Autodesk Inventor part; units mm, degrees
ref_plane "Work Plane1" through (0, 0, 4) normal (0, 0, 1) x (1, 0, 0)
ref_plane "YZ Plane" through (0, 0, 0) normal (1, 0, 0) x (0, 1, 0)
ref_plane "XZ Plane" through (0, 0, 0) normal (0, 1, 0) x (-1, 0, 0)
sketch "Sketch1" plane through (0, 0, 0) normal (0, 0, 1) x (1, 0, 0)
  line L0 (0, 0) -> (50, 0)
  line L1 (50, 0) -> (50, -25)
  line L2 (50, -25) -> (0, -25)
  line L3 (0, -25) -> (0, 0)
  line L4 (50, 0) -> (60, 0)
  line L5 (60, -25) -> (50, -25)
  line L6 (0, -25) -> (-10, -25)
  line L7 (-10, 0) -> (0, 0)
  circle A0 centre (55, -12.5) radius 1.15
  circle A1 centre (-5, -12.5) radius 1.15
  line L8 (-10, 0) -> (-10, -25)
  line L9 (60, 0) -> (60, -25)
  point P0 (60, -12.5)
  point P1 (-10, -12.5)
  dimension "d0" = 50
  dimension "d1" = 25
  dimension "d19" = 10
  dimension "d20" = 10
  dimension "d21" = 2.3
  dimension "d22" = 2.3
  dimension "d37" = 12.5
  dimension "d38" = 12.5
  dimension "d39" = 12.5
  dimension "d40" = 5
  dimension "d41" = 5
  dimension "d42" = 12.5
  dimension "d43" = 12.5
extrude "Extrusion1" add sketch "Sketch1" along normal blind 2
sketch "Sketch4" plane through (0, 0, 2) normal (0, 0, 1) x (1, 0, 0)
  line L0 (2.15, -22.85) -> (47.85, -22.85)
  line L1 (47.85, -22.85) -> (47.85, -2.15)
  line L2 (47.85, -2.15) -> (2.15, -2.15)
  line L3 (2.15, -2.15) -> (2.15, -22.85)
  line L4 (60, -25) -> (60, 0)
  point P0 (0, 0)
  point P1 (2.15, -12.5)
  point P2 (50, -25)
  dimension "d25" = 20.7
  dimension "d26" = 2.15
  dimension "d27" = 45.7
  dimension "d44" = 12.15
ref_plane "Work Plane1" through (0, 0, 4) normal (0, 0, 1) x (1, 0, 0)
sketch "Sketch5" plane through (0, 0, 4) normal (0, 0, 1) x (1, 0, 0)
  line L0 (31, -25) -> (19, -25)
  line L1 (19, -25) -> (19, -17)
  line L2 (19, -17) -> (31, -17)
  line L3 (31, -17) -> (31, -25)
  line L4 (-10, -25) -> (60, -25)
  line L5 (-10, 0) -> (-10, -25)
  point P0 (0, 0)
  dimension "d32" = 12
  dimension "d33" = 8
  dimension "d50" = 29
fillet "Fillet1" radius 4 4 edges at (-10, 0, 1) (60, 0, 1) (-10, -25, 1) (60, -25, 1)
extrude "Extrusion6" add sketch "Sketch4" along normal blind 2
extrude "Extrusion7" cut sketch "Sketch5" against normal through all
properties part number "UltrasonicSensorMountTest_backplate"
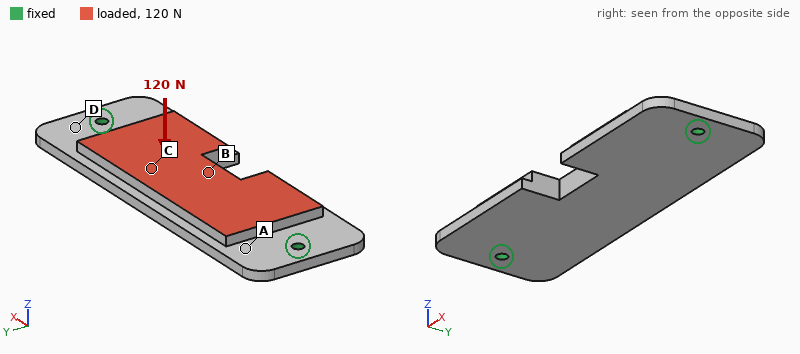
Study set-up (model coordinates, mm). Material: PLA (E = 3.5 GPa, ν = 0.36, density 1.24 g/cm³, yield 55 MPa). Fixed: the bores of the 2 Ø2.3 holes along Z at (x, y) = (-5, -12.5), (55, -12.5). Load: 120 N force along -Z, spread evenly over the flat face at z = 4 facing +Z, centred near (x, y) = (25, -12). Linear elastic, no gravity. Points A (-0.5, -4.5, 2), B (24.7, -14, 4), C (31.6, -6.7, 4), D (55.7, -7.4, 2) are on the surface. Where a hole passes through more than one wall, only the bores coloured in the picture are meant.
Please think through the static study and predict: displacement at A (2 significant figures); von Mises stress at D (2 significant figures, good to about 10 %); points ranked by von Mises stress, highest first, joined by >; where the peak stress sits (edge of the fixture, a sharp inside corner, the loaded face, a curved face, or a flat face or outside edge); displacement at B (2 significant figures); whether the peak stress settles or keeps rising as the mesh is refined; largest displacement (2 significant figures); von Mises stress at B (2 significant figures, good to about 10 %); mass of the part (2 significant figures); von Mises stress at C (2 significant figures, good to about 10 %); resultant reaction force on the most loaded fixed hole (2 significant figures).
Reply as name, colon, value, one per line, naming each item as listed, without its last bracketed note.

displacement at A: 0.16 mm
von Mises stress at D: 8.5 MPa
points ranked by von Mises stress, highest first, joined by >: B > C > D > A
where the peak stress sits: edge of the fixture
displacement at B: 0.61 mm
whether the peak stress settles or keeps rising as the mesh is refined: keeps rising
largest displacement: 0.67 mm
von Mises stress at B: 18 MPa
mass of the part: 6.2 g
von Mises stress at C: 14 MPa
resultant reaction force on the most loaded fixed hole: 130 N
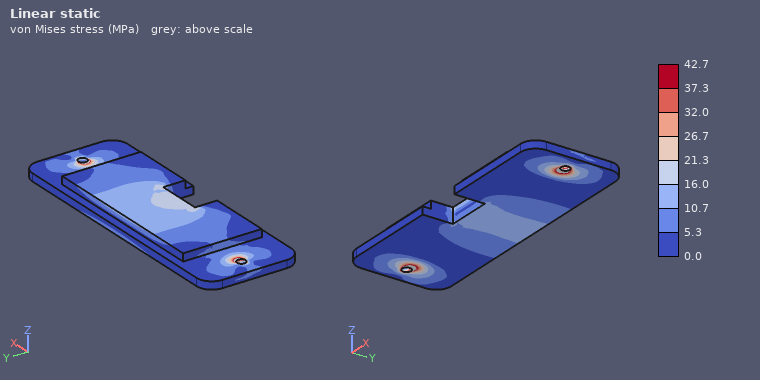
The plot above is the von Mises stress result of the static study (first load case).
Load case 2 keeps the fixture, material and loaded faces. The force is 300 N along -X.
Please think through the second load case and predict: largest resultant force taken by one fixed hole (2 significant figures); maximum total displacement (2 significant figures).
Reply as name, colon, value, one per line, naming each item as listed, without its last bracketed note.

largest resultant force taken by one fixed hole: 150 N
maximum total displacement: 34 µm
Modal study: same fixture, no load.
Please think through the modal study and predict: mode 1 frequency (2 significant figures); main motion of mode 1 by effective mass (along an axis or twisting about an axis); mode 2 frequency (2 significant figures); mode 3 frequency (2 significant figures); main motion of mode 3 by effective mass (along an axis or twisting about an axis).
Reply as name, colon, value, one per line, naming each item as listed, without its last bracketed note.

mode 1 frequency: 1100 Hz
main motion of mode 1 by effective mass: along Z
mode 2 frequency: 1400 Hz
mode 3 frequency: 2900 Hz
main motion of mode 3 by effective mass: twisting about Y
